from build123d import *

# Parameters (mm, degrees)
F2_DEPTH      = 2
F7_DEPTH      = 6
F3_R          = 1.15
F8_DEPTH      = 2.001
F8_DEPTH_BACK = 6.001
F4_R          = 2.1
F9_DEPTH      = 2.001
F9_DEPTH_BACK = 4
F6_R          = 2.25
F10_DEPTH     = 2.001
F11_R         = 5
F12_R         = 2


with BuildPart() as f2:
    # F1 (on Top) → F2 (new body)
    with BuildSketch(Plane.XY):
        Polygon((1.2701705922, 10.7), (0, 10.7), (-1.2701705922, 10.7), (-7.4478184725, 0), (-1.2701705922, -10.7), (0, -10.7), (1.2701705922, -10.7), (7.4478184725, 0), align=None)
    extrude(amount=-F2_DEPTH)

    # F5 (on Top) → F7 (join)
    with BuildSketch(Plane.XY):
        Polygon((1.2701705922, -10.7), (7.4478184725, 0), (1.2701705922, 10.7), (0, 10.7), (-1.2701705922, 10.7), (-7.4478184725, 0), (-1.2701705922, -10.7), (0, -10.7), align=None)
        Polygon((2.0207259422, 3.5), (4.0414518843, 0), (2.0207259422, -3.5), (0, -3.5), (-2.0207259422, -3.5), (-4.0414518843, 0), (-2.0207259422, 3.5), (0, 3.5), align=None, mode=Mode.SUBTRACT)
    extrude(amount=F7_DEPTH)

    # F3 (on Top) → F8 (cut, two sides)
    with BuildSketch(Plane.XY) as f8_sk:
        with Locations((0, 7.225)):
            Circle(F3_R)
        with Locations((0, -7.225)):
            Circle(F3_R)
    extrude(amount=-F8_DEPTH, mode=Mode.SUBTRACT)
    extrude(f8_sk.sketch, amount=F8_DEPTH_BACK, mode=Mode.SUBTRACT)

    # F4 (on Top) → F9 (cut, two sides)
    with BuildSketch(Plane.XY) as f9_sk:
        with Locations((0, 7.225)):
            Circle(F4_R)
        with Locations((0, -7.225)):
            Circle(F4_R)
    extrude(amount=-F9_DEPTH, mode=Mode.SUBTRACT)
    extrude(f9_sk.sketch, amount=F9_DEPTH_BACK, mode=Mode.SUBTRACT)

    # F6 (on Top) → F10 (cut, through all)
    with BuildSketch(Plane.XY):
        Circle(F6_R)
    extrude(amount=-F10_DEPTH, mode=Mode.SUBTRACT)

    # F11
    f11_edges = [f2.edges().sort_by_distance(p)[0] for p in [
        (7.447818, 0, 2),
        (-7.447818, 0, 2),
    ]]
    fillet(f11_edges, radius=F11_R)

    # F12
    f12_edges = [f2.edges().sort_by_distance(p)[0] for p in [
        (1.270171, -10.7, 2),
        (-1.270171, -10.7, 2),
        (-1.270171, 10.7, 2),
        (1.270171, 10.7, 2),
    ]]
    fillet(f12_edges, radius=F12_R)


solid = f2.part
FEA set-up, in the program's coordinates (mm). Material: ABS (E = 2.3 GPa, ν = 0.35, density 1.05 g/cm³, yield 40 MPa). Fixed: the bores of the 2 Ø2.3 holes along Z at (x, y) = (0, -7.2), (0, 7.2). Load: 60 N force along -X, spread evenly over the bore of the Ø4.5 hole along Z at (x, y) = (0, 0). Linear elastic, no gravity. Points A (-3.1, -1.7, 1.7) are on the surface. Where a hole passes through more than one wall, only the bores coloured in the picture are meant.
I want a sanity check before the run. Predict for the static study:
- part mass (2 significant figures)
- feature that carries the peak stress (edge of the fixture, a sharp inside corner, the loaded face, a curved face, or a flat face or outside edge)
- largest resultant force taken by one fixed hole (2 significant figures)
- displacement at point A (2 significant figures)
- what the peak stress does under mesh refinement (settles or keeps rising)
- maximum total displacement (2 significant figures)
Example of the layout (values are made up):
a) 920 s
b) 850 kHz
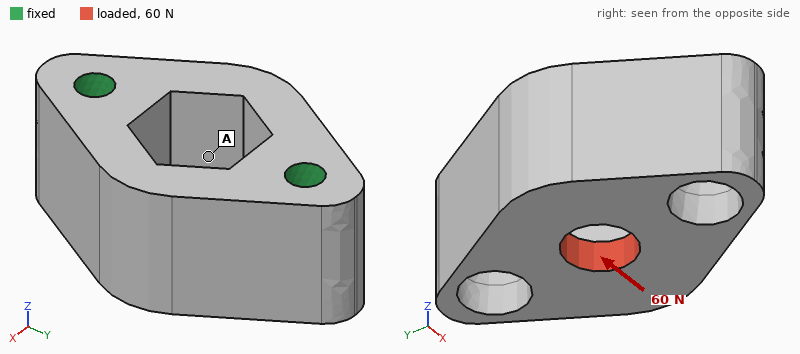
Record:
a) 1.0 g
b) edge of the fixture
c) 30 N
d) 0.051 mm
e) keeps rising
f) 0.11 mm
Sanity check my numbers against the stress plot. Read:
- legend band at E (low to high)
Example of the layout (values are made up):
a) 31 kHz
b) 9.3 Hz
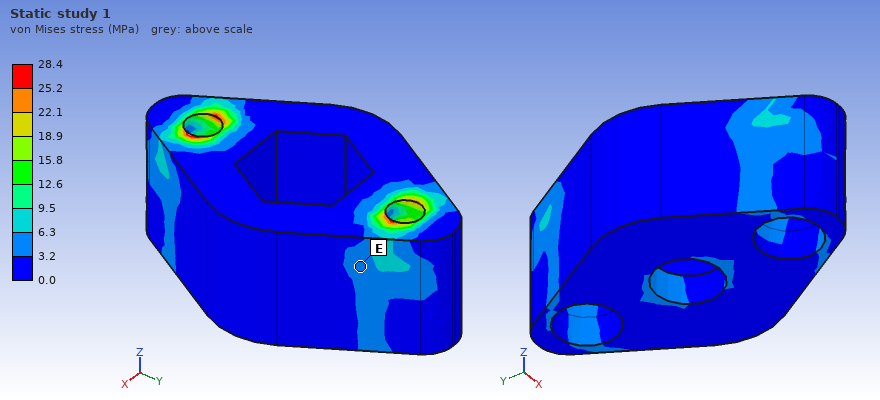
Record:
a) 3.2 to 6.3 MPa
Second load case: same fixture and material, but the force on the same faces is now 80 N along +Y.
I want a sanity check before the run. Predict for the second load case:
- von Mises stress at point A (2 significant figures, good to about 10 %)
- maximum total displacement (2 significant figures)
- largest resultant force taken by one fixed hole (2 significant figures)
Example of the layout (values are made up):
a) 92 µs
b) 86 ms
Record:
a) 2.4 MPa
b) 23 µm
c) 50 N
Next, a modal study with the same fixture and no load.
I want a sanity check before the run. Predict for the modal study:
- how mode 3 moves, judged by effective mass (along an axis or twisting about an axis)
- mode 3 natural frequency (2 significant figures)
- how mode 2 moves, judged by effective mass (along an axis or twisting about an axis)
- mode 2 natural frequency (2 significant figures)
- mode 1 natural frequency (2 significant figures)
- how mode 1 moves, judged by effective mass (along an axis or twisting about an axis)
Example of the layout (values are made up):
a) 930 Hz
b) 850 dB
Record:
a) along Y
b) 16 kHz
c) along Z
d) 14 kHz
e) 5500 Hz
f) along X
